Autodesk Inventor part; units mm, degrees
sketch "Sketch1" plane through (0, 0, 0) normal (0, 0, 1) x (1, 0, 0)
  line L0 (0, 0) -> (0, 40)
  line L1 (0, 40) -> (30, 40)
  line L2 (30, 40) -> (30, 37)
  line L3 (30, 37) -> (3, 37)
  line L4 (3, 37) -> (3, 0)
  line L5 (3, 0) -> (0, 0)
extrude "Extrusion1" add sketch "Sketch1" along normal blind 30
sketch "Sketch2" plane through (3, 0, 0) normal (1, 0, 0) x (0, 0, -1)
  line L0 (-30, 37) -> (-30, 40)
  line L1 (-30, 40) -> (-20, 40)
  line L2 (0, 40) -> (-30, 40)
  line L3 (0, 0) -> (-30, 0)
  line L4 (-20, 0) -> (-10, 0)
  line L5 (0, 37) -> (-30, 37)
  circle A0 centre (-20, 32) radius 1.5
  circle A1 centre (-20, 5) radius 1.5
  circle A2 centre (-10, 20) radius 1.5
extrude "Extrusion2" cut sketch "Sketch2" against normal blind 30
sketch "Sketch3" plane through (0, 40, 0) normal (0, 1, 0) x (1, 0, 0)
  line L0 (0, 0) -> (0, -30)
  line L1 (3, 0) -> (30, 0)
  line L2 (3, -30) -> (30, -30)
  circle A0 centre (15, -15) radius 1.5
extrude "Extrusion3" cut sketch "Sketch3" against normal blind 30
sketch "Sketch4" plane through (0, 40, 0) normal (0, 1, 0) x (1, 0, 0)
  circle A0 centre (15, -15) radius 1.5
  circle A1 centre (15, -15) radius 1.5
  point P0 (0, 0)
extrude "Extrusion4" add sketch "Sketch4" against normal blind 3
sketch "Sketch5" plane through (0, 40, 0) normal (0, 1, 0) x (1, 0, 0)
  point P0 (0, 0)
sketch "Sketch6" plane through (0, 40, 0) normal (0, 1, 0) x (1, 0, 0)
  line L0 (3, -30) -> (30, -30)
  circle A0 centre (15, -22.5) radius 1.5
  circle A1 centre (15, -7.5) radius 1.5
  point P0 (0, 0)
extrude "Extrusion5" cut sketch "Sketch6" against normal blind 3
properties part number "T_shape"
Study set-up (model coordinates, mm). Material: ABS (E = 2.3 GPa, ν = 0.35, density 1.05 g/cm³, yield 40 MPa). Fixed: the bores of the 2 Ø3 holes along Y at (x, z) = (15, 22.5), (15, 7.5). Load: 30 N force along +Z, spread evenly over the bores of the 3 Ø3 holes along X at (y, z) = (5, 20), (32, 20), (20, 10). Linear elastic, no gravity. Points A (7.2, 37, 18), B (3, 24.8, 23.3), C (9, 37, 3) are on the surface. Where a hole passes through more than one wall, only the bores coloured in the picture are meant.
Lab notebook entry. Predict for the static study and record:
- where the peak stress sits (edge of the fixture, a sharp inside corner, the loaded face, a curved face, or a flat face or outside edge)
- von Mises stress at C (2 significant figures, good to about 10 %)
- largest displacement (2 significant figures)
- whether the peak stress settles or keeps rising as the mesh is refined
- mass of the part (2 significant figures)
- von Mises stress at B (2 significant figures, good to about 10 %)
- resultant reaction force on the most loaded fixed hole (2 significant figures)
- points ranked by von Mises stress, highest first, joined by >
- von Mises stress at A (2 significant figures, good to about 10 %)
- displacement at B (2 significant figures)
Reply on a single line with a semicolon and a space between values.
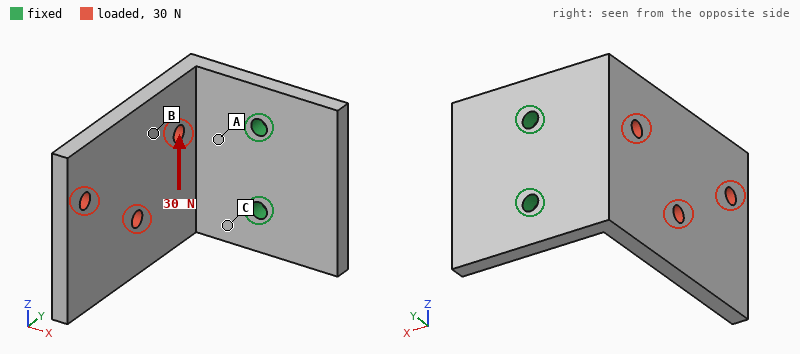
edge of the fixture; 4.8 MPa; 0.62 mm; keeps rising; 6.2 g; 1.5 MPa; 41 N; A > C > B; 6.4 MPa; 0.25 mm
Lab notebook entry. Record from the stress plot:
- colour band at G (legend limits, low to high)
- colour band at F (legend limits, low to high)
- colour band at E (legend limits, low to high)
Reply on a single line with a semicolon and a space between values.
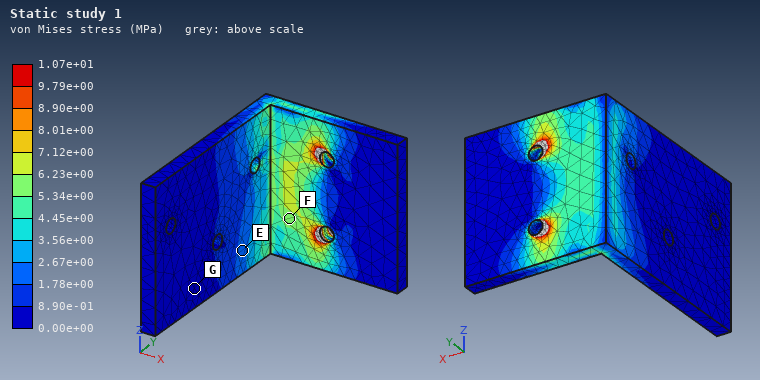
0.00e+00 to 8.90e-01 MPa; 5.34e+00 to 6.23e+00 MPa; 1.78e+00 to 2.67e+00 MPa
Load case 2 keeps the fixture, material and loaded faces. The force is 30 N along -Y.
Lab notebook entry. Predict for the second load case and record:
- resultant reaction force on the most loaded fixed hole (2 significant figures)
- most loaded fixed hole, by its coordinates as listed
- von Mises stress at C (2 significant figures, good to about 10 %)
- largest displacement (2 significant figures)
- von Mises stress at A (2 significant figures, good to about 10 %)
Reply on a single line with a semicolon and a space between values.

18 N; (15, 22.5); 4.3 MPa; 0.69 mm; 3.6 MPa
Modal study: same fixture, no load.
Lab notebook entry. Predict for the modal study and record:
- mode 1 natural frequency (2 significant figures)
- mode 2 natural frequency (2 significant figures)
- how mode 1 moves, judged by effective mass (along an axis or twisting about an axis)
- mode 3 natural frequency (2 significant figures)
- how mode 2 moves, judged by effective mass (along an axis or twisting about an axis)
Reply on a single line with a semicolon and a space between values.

320 Hz; 690 Hz; along X; 1300 Hz; along Z
